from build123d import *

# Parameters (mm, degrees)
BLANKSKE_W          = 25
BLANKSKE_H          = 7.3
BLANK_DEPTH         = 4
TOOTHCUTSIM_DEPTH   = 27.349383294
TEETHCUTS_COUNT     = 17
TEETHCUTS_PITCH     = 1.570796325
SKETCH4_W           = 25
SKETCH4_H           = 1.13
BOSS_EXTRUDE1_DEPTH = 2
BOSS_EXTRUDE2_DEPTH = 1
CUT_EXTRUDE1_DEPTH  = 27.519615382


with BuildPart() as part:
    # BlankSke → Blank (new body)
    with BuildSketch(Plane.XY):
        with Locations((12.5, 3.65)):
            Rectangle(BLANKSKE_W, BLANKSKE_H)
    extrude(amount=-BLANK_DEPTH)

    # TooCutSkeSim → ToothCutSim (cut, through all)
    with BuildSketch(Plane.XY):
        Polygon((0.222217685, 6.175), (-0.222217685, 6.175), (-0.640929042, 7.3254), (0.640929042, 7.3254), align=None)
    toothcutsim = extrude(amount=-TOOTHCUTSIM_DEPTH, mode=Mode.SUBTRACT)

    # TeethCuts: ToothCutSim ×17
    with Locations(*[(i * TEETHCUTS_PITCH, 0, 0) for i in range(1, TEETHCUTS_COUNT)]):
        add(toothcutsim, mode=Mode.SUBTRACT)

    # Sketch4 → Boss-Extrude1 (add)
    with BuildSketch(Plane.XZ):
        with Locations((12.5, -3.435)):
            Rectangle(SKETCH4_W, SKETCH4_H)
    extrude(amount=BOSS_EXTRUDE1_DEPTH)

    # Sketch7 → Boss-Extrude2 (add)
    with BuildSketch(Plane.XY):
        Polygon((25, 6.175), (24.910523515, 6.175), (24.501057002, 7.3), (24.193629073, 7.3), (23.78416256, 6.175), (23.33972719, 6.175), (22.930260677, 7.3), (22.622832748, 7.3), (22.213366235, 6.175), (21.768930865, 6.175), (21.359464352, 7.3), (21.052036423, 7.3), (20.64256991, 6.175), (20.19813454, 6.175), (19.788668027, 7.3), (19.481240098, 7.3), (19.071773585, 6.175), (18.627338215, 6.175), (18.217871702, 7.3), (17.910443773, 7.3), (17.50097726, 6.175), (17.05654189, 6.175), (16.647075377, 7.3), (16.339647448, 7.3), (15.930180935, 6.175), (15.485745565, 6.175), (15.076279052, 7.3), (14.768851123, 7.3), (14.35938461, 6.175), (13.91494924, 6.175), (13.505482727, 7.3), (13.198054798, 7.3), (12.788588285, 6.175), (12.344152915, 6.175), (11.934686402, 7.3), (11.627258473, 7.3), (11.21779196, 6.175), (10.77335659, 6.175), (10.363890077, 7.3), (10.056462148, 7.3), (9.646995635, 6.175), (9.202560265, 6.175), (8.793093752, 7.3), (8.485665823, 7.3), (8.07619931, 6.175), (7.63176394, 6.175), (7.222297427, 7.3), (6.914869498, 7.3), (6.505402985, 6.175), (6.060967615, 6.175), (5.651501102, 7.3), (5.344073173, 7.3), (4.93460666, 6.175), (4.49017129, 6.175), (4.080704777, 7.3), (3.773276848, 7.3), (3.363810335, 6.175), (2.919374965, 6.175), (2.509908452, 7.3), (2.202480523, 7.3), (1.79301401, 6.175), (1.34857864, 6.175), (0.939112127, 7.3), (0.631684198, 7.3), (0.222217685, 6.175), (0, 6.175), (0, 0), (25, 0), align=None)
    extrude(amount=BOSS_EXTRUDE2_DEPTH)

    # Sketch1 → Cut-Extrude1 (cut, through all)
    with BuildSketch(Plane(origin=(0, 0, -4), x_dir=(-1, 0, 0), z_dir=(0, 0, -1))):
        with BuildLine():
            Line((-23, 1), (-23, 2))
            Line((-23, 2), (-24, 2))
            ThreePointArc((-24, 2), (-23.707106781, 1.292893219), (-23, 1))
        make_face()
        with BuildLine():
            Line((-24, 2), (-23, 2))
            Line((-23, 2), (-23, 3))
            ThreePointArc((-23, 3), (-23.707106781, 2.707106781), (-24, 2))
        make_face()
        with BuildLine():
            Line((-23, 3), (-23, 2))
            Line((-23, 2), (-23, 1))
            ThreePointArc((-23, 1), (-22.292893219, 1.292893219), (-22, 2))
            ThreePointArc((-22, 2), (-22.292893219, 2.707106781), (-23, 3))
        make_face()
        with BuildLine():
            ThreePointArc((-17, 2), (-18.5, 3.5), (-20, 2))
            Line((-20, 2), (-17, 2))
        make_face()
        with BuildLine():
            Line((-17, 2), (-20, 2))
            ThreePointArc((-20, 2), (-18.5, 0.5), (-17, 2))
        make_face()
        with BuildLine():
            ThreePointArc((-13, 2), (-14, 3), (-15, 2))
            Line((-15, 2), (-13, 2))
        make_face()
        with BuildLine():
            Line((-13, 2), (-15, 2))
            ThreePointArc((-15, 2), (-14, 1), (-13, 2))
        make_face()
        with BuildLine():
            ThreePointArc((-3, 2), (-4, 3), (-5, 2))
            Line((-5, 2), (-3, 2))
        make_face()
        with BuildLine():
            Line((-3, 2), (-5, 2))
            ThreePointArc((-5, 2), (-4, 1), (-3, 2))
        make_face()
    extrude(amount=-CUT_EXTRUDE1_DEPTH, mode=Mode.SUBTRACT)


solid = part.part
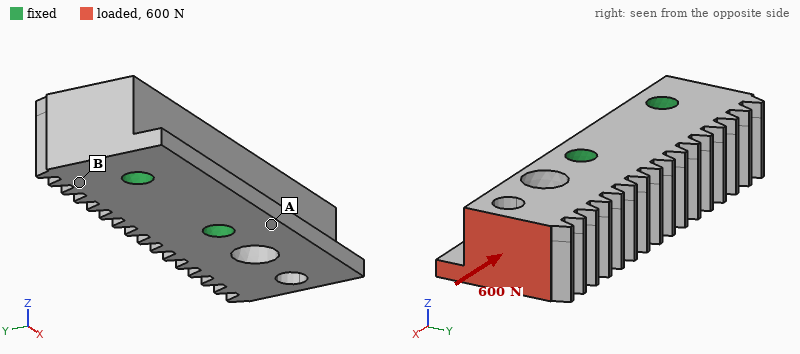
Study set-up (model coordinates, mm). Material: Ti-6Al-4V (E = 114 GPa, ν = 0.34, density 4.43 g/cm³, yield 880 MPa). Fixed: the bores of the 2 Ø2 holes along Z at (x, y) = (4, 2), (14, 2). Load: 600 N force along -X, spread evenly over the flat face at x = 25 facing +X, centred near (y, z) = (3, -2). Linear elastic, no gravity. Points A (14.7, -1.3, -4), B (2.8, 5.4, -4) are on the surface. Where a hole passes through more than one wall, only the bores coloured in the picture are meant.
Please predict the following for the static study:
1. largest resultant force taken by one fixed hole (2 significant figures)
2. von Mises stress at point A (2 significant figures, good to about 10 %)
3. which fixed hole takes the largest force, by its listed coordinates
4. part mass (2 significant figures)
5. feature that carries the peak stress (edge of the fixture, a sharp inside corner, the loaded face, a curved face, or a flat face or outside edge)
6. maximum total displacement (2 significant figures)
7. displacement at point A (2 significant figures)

510 N
20 MPa
(14, 2)
3.6 g
a curved face
3.9 µm
0.65 µm
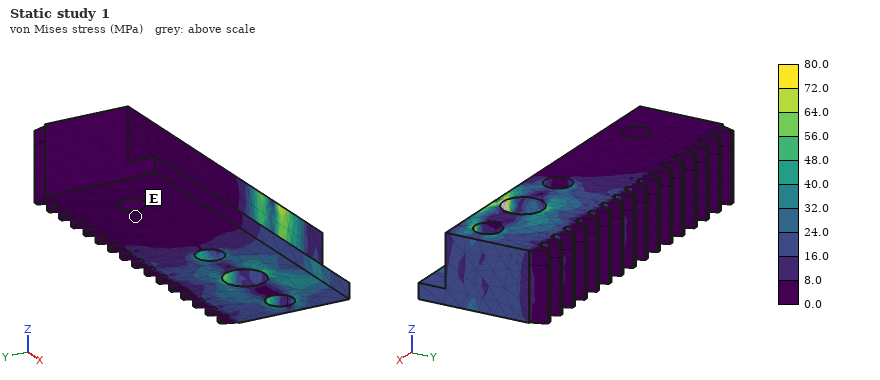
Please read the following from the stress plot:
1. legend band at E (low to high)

0.0 to 8.0 MPa
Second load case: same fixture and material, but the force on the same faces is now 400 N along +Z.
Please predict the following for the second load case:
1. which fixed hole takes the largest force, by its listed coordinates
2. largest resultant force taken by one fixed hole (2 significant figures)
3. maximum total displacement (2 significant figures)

(14, 2)
500 N
45 µm
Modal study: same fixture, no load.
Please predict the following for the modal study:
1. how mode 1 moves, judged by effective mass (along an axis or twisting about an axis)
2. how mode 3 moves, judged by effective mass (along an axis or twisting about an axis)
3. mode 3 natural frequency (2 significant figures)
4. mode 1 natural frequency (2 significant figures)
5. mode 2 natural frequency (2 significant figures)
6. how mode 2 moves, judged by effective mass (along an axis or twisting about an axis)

along Z
twisting about X
46 kHz
25 kHz
28 kHz
along Y
